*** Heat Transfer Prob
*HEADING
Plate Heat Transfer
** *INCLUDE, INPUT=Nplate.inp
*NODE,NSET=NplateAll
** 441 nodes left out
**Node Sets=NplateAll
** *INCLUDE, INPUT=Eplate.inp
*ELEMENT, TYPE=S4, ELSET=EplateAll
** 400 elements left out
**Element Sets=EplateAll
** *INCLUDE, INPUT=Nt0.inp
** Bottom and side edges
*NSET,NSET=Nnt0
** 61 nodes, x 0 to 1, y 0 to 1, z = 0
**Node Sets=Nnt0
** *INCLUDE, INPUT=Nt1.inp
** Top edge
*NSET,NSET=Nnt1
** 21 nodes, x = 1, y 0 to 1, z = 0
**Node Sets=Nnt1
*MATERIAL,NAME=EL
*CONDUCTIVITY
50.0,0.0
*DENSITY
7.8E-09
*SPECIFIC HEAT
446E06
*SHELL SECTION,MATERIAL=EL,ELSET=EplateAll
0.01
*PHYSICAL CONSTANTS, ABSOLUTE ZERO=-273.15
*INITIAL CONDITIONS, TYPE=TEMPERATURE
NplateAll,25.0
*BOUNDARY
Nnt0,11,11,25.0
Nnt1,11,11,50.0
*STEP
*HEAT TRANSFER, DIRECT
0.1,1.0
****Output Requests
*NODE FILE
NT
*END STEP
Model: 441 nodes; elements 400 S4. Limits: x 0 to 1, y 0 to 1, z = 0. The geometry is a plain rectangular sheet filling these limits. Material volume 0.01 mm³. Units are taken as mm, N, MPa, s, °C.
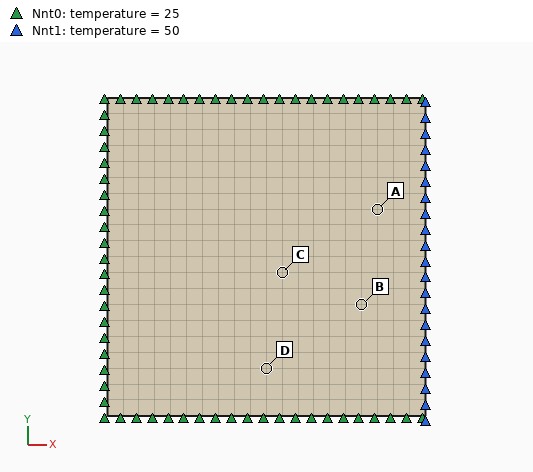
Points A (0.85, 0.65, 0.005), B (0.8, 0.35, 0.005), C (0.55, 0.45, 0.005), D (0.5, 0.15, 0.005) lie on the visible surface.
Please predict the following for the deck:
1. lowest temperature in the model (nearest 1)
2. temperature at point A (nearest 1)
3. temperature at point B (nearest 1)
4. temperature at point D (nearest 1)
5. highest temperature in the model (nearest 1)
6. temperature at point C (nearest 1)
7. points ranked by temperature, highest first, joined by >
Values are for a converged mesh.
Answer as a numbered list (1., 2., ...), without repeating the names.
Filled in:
1. 25 °C
2. 42 °C
3. 40 °C
4. 28 °C
5. 50 °C
6. 32 °C
7. A > B > C > D
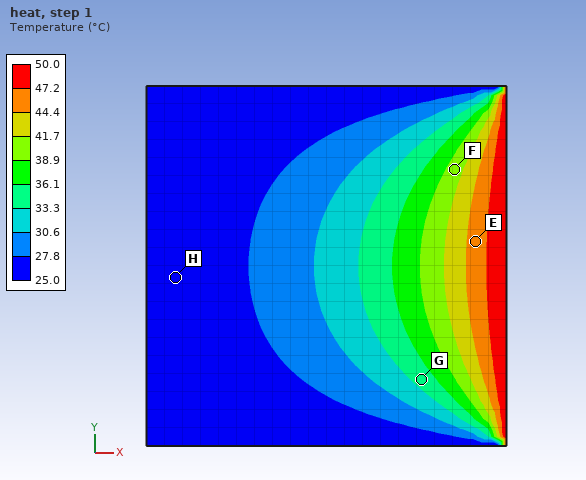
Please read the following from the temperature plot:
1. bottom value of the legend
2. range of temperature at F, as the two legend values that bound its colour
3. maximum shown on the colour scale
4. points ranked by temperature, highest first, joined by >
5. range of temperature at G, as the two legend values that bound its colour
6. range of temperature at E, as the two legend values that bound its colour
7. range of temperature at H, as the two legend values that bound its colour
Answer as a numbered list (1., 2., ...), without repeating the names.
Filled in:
1. 25.0 °C
2. 38.9 to 41.7 °C
3. 50.0 °C
4. E > F > G > H
5. 33.3 to 36.1 °C
6. 44.4 to 47.2 °C
7. 25.0 to 27.8 °C
